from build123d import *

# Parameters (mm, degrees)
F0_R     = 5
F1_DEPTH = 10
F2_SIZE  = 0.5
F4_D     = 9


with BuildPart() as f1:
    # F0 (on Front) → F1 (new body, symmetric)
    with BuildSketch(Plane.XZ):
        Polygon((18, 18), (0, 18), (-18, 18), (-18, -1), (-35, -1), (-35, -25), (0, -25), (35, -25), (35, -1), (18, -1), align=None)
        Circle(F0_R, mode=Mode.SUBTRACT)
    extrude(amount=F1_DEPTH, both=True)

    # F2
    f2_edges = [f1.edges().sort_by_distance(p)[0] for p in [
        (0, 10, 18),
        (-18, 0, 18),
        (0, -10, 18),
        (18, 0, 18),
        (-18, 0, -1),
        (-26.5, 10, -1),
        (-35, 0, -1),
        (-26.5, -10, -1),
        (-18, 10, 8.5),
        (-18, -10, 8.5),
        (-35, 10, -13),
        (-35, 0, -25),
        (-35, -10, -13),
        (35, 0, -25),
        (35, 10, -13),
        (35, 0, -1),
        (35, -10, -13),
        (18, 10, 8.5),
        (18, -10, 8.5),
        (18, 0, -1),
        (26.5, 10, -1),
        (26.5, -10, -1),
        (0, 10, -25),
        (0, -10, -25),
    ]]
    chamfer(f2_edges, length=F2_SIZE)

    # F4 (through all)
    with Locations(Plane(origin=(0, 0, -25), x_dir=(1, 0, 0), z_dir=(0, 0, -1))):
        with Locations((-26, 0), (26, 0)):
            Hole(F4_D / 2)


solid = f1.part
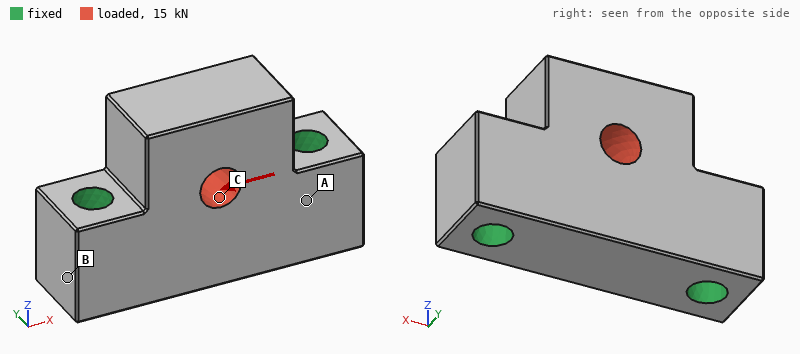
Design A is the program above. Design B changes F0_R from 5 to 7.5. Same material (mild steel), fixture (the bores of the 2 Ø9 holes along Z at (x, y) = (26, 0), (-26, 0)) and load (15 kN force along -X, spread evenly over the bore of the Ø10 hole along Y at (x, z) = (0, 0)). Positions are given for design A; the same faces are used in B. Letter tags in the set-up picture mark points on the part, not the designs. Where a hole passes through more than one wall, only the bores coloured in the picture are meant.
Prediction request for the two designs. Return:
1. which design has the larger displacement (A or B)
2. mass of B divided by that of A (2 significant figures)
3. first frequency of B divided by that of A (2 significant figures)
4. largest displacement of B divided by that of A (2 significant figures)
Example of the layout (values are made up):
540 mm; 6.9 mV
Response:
B; 0.95; 1.0; 1.3
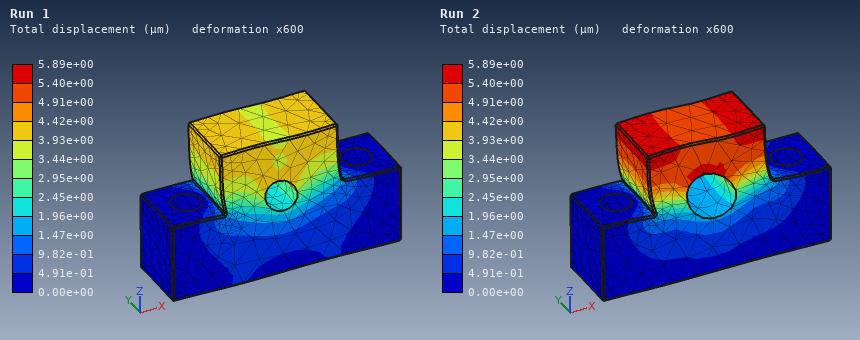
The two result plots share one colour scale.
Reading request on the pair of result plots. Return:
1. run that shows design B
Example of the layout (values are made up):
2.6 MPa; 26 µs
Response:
Run 2
